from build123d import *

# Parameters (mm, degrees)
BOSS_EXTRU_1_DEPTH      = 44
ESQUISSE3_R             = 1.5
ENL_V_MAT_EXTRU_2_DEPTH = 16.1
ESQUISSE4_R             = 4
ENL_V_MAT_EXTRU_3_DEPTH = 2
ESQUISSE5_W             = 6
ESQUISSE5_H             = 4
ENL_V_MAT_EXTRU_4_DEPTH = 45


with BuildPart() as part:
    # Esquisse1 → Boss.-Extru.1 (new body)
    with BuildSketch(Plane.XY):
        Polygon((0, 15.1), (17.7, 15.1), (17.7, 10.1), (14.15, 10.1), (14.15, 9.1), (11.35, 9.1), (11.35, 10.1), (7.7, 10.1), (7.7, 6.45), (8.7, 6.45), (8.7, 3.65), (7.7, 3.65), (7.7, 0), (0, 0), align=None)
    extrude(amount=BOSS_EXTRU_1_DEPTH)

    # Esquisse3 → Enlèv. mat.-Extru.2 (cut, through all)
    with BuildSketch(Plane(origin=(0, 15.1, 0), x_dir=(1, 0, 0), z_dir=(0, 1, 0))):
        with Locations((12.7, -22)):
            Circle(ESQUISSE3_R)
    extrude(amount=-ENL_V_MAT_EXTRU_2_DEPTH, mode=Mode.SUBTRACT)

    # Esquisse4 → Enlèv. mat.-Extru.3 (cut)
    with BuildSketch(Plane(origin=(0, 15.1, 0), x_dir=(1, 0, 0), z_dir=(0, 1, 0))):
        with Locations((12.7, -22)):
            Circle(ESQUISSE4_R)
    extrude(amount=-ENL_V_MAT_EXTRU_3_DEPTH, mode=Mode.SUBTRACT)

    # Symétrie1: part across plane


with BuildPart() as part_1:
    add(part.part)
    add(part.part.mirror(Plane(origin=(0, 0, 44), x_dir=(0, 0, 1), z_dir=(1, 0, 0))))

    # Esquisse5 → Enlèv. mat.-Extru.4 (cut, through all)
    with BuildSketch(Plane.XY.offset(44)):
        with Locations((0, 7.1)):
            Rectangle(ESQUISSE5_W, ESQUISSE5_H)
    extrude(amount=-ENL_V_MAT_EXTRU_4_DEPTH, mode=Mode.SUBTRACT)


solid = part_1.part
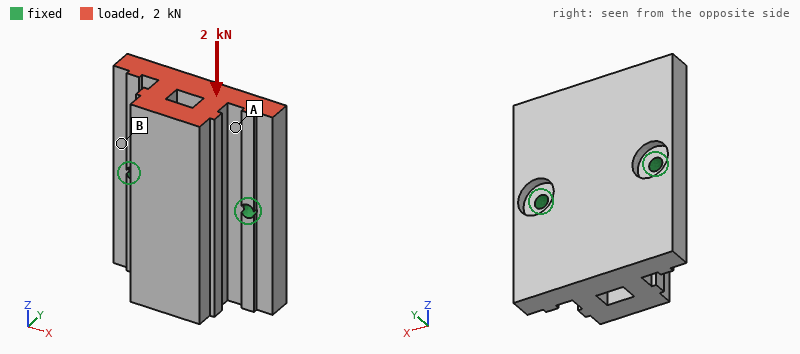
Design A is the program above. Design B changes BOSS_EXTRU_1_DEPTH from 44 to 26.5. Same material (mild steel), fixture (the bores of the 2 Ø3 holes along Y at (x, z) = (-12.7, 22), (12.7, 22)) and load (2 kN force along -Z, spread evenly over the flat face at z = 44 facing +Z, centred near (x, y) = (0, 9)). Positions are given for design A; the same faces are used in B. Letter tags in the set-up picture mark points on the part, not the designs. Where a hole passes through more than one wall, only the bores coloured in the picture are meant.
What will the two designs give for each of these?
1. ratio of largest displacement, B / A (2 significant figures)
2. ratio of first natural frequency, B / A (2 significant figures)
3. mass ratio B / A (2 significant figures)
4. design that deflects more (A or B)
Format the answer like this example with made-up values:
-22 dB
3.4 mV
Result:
1.5
1.2
0.59
B
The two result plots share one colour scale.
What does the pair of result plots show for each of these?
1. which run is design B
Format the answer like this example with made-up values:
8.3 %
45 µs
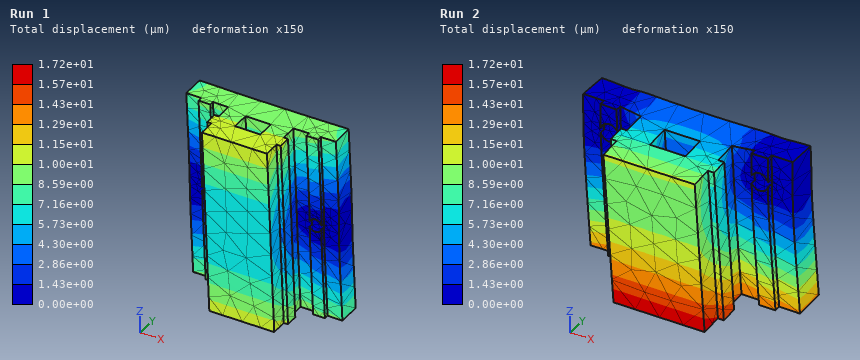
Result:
Run 2
